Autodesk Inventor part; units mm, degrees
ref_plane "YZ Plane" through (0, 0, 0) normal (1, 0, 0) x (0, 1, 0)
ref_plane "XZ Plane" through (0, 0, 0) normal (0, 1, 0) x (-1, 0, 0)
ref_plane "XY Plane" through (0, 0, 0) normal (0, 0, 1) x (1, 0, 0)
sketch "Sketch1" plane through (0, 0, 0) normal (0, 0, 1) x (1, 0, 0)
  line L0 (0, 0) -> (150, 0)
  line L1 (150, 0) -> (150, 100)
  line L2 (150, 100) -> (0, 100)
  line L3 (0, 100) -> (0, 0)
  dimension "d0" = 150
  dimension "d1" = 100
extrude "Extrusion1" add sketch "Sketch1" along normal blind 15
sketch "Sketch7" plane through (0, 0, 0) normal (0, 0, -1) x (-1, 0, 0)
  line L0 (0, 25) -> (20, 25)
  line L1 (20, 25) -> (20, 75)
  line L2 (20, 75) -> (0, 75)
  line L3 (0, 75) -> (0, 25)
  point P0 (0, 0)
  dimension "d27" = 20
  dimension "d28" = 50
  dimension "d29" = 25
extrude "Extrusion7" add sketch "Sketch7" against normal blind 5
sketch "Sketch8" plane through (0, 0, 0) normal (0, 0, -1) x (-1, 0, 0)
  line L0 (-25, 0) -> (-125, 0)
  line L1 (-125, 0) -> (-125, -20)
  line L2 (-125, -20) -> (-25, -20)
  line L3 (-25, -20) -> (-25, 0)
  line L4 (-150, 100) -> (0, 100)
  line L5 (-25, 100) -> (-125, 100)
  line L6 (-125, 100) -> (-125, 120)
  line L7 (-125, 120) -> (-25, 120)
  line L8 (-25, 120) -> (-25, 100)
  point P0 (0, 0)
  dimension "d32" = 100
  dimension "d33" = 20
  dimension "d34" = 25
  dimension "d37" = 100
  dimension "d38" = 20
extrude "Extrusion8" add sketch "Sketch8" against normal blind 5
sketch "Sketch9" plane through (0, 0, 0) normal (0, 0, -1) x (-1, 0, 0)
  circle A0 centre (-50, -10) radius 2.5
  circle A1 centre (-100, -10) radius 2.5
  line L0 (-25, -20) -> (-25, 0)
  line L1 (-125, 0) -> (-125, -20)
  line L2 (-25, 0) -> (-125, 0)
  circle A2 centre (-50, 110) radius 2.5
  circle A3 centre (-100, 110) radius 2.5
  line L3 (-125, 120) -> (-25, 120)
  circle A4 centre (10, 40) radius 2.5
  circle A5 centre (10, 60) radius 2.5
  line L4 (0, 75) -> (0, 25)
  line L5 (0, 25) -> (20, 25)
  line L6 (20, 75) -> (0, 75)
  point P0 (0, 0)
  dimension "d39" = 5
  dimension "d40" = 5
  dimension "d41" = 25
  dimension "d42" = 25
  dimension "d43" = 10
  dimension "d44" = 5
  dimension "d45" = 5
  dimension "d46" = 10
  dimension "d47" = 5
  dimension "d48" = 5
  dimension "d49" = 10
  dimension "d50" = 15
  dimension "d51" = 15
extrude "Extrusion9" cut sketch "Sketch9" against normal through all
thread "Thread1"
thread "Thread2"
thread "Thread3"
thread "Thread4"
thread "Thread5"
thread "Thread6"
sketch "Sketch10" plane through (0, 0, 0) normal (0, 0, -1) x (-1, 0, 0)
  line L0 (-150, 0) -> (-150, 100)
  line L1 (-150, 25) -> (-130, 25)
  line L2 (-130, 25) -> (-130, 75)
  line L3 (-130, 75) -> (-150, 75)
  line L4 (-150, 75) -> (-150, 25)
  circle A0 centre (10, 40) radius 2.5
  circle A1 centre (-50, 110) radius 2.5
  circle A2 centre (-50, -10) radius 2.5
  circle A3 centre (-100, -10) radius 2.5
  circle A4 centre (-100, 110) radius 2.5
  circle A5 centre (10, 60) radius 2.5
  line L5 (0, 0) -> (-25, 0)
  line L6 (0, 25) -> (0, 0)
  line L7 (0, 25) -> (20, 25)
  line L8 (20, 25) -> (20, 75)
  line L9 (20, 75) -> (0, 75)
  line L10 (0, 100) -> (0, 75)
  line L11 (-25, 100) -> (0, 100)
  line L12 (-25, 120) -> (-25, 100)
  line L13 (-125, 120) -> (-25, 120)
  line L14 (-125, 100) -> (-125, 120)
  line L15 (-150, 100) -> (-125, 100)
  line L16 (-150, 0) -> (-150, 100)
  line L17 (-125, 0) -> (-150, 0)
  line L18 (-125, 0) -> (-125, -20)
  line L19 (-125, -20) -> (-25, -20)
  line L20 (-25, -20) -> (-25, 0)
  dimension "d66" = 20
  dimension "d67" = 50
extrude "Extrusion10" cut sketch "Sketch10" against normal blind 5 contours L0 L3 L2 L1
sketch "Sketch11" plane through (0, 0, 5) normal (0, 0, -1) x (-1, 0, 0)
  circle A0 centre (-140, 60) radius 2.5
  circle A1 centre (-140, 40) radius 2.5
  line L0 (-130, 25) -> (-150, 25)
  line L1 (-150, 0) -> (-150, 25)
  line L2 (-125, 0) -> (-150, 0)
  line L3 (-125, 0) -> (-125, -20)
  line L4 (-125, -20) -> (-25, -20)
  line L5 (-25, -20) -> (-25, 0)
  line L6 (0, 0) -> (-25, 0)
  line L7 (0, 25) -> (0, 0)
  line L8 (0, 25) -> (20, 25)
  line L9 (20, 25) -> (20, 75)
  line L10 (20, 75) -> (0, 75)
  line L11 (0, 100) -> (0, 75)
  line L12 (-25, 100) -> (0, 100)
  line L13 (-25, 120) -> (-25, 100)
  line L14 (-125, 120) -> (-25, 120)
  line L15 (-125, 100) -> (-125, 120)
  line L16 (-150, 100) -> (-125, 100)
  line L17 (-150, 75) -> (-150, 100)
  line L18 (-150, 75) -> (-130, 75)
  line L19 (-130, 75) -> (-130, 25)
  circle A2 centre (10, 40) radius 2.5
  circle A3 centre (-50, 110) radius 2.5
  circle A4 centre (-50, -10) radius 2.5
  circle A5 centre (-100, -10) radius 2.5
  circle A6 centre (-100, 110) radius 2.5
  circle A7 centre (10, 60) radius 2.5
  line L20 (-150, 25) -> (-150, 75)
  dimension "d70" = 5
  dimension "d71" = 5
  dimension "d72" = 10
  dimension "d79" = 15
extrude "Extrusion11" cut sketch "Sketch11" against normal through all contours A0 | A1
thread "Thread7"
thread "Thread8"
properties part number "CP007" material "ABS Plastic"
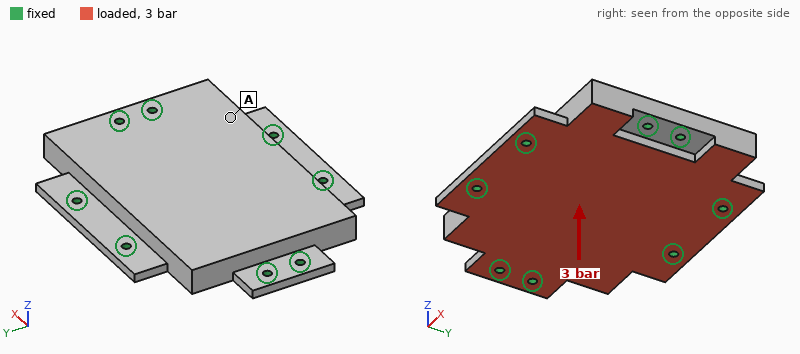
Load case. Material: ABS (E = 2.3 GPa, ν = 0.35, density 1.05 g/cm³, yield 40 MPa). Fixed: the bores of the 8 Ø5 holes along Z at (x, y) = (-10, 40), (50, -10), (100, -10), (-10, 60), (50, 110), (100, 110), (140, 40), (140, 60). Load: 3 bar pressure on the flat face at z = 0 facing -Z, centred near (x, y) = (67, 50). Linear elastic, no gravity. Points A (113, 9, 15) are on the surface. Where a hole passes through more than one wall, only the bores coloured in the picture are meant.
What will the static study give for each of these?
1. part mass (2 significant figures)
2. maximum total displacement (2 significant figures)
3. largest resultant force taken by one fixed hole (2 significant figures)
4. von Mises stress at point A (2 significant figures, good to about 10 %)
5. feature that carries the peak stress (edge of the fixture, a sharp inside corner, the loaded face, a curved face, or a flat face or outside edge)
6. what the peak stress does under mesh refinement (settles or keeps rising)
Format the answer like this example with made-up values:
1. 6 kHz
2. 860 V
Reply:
1. 260 g
2. 0.54 mm
3. 1.1 kN
4. 4.5 MPa
5. edge of the fixture
6. keeps rising
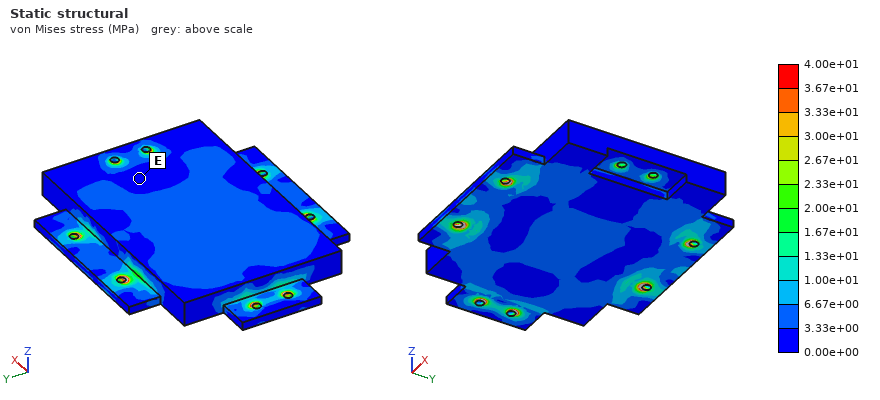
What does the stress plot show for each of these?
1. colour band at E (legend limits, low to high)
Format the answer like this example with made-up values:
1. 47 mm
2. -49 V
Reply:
1. 0.00e+00 to 3.33e+00 MPa
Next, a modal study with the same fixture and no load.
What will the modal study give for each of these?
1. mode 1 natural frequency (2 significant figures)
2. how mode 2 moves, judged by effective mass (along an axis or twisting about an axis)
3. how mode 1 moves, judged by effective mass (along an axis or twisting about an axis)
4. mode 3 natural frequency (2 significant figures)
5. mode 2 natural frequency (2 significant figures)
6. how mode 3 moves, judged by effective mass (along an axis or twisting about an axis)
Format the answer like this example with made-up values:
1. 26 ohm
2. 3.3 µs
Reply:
1. 1100 Hz
2. twisting about X
3. along Z
4. 1700 Hz
5. 1500 Hz
6. twisting about Y
